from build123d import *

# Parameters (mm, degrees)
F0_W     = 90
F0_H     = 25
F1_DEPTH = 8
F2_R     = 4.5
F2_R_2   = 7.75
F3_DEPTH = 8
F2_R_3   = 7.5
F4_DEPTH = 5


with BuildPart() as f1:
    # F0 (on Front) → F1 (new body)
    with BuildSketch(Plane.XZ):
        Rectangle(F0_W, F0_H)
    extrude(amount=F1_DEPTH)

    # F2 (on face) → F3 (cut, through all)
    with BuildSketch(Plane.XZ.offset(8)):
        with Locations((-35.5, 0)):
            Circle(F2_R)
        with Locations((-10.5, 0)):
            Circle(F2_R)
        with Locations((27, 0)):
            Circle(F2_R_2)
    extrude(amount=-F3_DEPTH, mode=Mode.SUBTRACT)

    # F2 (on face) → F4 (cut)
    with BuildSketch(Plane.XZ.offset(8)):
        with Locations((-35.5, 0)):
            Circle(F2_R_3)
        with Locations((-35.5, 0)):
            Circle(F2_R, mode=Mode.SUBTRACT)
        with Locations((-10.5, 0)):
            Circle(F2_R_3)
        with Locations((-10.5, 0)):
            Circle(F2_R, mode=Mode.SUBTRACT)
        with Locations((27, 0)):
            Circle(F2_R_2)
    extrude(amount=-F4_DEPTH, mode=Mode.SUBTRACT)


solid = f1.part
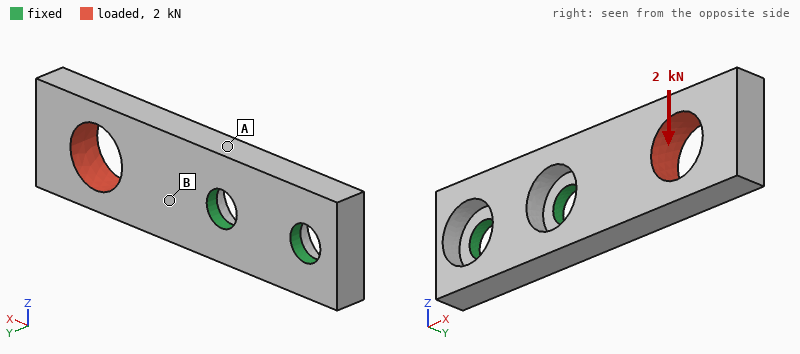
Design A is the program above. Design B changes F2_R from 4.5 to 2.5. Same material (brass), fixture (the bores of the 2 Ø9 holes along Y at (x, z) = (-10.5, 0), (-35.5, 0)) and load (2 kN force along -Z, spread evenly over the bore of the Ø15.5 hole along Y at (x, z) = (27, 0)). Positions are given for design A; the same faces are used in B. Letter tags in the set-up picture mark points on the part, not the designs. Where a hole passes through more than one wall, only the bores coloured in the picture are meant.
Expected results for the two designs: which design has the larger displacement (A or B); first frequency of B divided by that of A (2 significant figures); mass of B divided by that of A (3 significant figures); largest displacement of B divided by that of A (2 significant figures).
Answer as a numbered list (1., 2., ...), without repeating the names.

1. B
2. 0.89
3. 1.02
4. 1.3
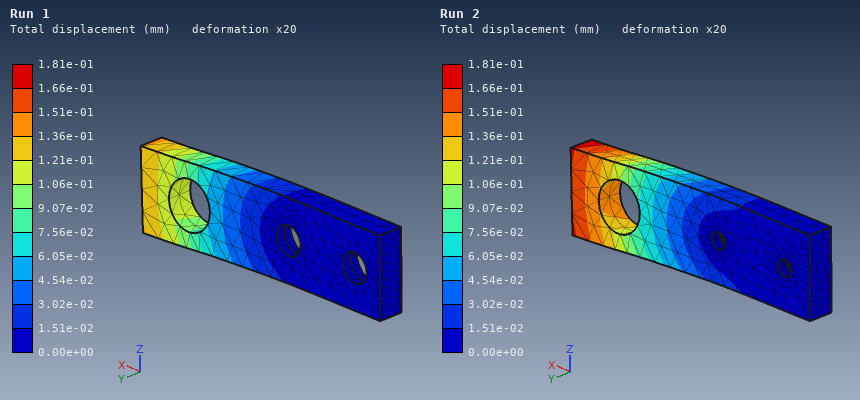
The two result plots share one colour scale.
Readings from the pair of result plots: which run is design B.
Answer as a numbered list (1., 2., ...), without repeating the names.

1. Run 2
